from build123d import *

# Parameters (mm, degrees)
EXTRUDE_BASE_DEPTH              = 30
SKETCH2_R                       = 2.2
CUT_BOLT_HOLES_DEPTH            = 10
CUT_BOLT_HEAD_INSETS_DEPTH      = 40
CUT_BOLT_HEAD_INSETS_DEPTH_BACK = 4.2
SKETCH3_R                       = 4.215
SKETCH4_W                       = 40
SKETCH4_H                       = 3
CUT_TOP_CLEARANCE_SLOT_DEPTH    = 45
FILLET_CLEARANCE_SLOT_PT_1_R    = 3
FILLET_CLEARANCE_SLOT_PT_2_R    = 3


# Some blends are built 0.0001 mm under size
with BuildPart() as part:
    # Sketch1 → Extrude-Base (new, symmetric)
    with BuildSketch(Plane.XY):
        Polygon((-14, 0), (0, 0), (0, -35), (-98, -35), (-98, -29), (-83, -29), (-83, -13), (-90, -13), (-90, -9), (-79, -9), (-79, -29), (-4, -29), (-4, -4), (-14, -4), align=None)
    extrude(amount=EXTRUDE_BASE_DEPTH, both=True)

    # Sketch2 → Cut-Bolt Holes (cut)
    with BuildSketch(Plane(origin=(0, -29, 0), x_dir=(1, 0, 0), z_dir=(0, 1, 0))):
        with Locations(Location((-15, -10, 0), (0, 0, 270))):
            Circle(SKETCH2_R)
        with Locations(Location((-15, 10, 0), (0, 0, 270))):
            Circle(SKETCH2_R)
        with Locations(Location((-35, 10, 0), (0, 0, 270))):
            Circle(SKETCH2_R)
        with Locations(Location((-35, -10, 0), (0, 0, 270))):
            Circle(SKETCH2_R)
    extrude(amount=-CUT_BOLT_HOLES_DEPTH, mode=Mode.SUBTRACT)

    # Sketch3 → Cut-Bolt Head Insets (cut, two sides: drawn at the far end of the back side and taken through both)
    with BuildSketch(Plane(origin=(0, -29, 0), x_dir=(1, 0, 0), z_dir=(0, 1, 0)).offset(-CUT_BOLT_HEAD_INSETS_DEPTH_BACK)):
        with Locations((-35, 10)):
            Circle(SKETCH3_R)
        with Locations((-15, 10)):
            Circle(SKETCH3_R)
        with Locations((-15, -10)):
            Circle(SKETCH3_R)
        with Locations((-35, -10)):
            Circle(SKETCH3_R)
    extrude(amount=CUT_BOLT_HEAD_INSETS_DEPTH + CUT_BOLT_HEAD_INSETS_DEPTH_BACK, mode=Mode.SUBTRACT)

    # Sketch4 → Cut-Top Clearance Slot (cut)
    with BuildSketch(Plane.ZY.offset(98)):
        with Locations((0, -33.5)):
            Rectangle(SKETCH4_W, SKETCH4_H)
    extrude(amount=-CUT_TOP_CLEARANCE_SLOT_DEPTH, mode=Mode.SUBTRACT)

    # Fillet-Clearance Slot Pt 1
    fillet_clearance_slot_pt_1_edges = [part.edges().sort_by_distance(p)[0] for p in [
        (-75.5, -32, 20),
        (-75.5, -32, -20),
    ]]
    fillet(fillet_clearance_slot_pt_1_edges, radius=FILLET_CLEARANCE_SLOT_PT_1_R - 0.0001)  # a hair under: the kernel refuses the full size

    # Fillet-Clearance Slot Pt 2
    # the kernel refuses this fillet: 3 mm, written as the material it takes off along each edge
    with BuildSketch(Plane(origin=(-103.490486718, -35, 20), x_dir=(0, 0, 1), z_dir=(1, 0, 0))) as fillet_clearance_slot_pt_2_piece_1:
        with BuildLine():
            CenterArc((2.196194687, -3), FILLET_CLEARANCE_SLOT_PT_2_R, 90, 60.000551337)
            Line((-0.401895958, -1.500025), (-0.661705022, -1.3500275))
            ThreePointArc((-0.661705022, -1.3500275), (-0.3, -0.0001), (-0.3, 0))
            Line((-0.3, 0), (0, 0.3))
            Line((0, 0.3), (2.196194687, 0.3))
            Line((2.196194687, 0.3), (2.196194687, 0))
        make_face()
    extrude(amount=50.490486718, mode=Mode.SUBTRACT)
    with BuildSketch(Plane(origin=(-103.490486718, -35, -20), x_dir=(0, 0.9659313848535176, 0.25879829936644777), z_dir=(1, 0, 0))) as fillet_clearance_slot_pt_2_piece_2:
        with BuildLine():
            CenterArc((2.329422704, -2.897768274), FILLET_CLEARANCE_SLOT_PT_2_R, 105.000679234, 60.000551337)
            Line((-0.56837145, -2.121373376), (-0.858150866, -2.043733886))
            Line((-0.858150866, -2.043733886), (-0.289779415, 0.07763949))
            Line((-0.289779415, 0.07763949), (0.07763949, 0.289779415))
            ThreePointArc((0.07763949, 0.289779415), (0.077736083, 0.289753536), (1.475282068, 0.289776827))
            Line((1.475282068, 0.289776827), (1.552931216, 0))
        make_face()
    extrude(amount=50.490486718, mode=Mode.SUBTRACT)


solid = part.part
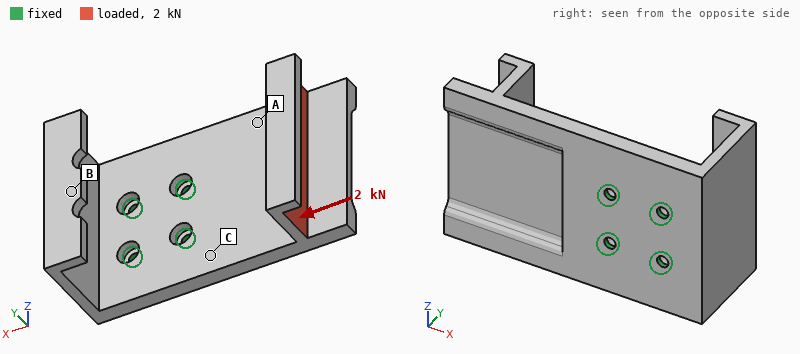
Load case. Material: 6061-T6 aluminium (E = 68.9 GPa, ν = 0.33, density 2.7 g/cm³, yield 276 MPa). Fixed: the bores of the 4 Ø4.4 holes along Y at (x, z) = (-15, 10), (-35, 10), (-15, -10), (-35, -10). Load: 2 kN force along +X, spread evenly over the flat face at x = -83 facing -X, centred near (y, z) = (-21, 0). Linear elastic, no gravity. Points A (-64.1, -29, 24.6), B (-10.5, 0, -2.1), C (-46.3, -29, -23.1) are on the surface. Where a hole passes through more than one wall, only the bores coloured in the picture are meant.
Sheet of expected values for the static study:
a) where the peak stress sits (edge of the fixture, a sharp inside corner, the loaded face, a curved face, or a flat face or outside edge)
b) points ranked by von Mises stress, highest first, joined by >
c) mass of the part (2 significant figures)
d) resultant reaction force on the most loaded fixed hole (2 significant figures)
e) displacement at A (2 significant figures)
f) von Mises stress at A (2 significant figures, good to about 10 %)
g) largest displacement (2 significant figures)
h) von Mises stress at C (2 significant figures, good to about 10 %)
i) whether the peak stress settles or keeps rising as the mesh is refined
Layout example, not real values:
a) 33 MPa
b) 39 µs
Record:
a) edge of the fixture
b) A > C > B
c) 120 g
d) 1.1 kN
e) 0.22 mm
f) 99 MPa
g) 1.0 mm
h) 75 MPa
i) keeps rising
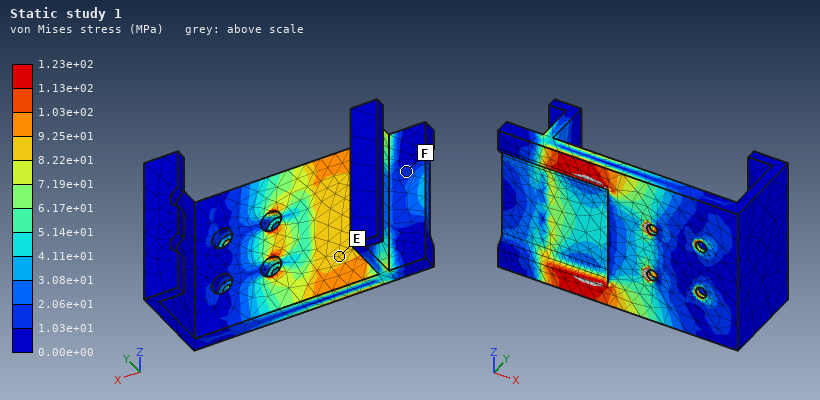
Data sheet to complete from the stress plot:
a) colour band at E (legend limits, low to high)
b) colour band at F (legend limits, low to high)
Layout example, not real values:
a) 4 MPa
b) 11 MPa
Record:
a) 8.22e+01 to 9.25e+01 MPa
b) 1.03e+01 to 2.06e+01 MPa
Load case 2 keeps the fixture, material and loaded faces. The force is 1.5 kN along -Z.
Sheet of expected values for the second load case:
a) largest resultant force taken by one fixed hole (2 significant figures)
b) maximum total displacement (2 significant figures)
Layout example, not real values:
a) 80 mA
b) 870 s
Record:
a) 2.2 kN
b) 0.31 mm
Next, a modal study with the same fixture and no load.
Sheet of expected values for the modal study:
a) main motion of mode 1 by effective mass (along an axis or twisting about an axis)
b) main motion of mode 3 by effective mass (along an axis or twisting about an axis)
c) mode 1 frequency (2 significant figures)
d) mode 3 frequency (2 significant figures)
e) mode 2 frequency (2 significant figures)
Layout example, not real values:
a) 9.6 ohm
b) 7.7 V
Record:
a) along Y
b) along X
c) 800 Hz
d) 1800 Hz
e) 1500 Hz
